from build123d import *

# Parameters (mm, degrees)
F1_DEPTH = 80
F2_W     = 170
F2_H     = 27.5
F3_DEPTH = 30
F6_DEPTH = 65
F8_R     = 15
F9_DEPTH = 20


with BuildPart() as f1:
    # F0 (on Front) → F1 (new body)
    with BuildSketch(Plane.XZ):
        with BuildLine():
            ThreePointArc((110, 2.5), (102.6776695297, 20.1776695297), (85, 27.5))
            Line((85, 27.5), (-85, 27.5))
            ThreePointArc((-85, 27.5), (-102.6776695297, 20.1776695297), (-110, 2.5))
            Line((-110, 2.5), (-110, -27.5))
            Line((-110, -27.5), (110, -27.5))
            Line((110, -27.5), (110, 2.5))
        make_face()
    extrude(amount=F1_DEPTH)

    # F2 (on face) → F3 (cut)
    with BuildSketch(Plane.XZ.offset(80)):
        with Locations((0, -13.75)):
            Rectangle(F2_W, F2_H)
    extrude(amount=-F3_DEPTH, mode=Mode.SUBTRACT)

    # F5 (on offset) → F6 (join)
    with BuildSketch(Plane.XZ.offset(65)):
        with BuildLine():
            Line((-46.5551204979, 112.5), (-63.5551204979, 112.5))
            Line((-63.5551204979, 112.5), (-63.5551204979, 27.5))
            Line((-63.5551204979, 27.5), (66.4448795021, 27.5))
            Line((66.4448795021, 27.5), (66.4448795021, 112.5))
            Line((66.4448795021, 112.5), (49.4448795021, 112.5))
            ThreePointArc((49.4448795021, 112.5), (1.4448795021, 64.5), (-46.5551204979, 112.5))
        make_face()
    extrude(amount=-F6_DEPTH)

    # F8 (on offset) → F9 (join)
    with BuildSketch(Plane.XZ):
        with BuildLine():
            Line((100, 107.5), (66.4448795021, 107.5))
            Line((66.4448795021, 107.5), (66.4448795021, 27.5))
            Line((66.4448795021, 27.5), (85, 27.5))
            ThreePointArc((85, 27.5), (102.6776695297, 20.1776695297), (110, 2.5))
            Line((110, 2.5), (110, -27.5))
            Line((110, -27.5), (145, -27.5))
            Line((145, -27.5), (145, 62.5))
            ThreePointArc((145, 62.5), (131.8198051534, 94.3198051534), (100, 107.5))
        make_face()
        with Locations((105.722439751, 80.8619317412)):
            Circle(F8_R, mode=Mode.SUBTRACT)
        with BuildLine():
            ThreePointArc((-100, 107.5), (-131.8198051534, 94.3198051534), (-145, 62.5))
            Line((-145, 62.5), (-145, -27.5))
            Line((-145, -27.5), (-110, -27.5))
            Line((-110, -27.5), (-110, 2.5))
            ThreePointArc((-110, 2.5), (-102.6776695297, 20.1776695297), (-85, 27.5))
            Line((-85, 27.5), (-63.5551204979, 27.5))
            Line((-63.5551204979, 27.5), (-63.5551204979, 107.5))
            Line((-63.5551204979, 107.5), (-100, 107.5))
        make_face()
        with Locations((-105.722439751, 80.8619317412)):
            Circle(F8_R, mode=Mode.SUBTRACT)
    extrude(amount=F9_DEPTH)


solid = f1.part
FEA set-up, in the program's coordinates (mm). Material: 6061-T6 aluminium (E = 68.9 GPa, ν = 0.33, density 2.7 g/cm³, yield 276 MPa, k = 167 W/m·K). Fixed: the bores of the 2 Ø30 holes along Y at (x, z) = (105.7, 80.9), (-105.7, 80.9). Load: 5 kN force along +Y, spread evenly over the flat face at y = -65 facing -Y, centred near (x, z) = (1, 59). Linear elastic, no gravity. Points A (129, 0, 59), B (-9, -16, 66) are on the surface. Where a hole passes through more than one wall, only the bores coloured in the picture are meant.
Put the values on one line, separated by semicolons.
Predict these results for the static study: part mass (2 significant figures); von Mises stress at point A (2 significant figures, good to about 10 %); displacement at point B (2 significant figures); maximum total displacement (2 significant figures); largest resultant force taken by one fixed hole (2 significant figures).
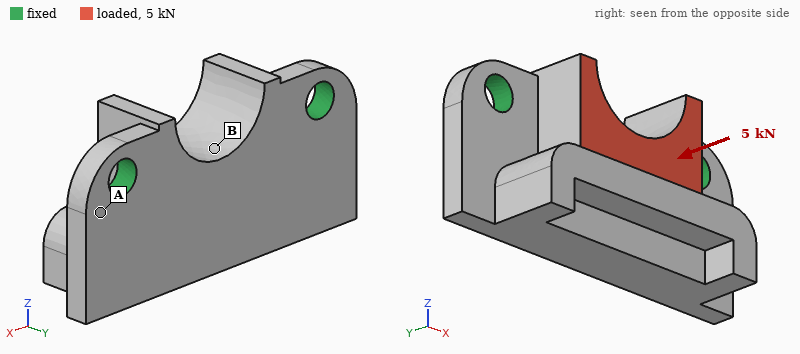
4.3 kg; 3.4 MPa; 9.2 µm; 19 µm; 2.7 kN
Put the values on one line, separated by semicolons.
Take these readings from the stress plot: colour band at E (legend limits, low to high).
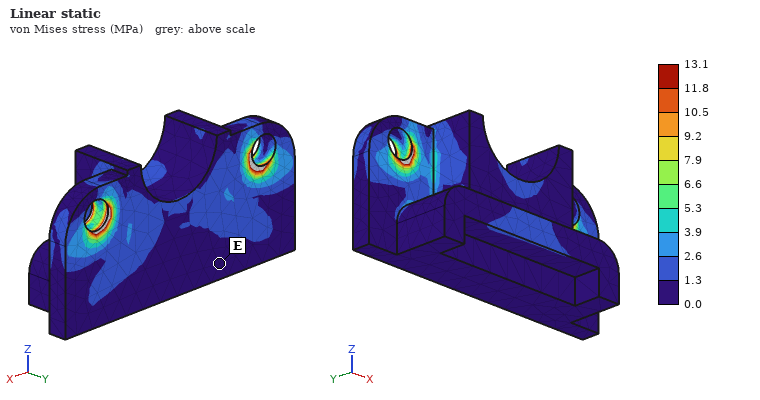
0.0 to 1.3 MPa
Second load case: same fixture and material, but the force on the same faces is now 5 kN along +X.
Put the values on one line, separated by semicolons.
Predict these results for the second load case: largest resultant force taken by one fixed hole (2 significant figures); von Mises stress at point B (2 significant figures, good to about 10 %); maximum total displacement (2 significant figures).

3.0 kN; 1.9 MPa; 9.3 µm
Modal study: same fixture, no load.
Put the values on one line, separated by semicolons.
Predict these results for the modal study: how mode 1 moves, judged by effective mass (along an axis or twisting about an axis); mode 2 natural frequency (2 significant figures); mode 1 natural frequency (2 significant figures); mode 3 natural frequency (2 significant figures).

along Y; 2300 Hz; 830 Hz; 3000 Hz
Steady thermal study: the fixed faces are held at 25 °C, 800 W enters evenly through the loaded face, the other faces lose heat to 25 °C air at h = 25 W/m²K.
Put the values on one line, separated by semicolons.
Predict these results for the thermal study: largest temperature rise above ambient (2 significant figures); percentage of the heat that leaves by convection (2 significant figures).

75 K; 16 %
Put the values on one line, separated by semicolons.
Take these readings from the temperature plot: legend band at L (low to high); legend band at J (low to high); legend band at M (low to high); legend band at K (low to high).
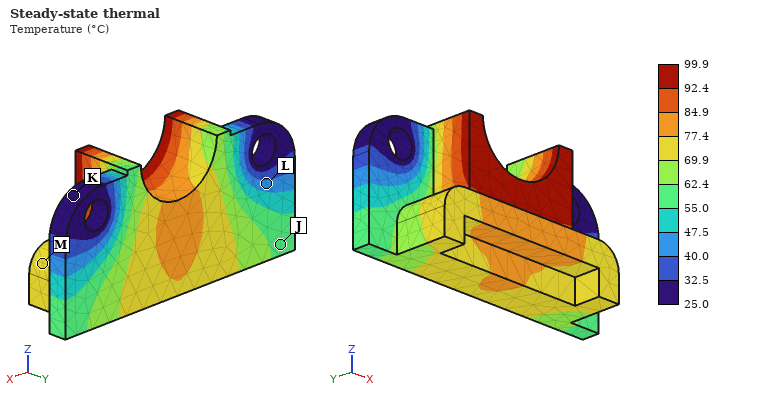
40.0 to 47.5 °C; 55.0 to 62.4 °C; 69.9 to 77.4 °C; 25.0 to 32.5 °C
